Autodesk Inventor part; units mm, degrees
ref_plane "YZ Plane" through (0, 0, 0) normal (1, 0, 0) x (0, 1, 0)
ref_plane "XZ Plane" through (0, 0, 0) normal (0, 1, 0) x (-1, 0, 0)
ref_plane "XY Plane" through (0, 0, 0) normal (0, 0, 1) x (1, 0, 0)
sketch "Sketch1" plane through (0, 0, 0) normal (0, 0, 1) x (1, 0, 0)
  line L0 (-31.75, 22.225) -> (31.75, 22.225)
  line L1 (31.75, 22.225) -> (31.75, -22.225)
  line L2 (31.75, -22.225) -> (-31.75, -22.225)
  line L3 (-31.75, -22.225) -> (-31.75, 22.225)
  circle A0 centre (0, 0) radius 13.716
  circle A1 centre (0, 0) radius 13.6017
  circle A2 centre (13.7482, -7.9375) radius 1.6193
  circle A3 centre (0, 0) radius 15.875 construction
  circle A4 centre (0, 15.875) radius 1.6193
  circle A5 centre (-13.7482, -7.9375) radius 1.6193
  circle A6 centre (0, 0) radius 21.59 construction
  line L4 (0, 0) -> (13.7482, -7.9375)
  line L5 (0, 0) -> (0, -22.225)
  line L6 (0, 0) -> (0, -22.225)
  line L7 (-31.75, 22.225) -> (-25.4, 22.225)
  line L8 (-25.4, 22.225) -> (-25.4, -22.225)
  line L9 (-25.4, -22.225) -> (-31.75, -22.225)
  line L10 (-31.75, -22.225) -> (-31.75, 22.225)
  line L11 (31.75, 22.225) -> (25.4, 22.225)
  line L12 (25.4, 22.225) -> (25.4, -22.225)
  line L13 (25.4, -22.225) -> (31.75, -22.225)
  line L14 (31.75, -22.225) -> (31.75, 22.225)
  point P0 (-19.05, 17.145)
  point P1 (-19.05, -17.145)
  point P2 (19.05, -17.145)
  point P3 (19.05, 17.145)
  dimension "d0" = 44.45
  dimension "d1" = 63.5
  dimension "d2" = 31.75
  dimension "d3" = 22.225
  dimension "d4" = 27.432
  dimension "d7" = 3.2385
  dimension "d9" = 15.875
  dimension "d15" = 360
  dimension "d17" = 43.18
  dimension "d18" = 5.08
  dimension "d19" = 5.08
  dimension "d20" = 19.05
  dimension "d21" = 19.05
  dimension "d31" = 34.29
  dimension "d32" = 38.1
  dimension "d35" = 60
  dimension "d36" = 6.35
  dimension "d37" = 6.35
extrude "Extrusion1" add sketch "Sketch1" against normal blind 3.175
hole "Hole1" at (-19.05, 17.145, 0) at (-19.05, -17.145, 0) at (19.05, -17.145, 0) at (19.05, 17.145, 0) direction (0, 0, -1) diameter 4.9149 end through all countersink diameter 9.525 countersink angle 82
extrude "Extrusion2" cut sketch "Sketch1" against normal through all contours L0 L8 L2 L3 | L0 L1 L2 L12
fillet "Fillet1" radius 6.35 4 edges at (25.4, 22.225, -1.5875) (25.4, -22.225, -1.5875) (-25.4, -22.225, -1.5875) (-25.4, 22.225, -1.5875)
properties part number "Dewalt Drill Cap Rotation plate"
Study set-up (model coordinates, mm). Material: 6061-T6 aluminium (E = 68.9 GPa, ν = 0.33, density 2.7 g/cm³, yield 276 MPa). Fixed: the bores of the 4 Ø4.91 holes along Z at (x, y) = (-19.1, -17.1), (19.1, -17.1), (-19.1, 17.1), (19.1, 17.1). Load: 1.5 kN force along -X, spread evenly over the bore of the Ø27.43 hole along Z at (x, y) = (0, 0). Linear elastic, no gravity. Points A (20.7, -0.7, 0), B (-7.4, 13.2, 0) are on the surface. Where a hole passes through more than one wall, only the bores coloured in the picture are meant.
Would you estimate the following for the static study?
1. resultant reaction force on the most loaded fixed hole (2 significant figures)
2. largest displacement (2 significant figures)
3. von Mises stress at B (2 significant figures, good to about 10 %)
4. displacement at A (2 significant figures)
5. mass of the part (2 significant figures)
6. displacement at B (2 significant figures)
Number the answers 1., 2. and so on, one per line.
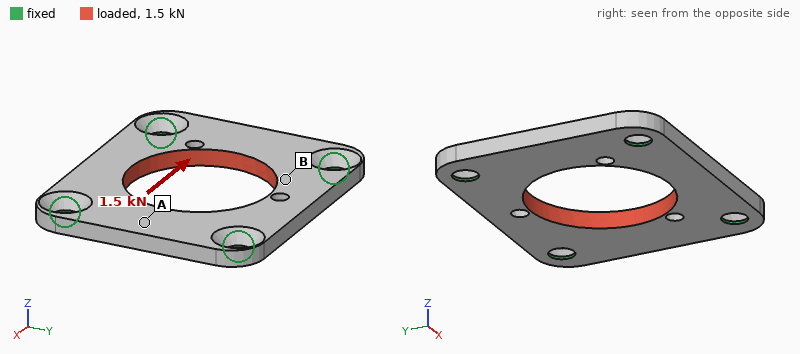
1. 380 N
2. 7.8 µm
3. 12 MPa
4. 6.4 µm
5. 12 g
6. 4.4 µm
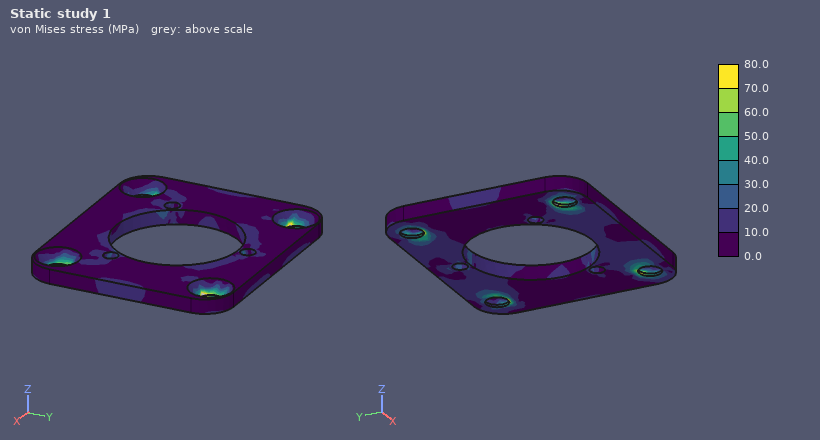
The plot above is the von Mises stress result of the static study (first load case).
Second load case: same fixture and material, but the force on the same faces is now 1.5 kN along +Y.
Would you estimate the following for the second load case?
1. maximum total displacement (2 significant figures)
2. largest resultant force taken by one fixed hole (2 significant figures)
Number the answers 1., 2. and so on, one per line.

1. 9.8 µm
2. 380 N
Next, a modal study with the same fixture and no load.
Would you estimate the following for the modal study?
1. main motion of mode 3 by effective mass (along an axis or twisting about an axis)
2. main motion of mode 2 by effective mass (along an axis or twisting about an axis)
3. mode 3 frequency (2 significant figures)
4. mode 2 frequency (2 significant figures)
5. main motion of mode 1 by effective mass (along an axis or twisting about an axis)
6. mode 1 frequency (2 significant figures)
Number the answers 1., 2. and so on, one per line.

1. along Z
2. twisting about X
3. 11 kHz
4. 10 kHz
5. along Z
6. 9500 Hz
